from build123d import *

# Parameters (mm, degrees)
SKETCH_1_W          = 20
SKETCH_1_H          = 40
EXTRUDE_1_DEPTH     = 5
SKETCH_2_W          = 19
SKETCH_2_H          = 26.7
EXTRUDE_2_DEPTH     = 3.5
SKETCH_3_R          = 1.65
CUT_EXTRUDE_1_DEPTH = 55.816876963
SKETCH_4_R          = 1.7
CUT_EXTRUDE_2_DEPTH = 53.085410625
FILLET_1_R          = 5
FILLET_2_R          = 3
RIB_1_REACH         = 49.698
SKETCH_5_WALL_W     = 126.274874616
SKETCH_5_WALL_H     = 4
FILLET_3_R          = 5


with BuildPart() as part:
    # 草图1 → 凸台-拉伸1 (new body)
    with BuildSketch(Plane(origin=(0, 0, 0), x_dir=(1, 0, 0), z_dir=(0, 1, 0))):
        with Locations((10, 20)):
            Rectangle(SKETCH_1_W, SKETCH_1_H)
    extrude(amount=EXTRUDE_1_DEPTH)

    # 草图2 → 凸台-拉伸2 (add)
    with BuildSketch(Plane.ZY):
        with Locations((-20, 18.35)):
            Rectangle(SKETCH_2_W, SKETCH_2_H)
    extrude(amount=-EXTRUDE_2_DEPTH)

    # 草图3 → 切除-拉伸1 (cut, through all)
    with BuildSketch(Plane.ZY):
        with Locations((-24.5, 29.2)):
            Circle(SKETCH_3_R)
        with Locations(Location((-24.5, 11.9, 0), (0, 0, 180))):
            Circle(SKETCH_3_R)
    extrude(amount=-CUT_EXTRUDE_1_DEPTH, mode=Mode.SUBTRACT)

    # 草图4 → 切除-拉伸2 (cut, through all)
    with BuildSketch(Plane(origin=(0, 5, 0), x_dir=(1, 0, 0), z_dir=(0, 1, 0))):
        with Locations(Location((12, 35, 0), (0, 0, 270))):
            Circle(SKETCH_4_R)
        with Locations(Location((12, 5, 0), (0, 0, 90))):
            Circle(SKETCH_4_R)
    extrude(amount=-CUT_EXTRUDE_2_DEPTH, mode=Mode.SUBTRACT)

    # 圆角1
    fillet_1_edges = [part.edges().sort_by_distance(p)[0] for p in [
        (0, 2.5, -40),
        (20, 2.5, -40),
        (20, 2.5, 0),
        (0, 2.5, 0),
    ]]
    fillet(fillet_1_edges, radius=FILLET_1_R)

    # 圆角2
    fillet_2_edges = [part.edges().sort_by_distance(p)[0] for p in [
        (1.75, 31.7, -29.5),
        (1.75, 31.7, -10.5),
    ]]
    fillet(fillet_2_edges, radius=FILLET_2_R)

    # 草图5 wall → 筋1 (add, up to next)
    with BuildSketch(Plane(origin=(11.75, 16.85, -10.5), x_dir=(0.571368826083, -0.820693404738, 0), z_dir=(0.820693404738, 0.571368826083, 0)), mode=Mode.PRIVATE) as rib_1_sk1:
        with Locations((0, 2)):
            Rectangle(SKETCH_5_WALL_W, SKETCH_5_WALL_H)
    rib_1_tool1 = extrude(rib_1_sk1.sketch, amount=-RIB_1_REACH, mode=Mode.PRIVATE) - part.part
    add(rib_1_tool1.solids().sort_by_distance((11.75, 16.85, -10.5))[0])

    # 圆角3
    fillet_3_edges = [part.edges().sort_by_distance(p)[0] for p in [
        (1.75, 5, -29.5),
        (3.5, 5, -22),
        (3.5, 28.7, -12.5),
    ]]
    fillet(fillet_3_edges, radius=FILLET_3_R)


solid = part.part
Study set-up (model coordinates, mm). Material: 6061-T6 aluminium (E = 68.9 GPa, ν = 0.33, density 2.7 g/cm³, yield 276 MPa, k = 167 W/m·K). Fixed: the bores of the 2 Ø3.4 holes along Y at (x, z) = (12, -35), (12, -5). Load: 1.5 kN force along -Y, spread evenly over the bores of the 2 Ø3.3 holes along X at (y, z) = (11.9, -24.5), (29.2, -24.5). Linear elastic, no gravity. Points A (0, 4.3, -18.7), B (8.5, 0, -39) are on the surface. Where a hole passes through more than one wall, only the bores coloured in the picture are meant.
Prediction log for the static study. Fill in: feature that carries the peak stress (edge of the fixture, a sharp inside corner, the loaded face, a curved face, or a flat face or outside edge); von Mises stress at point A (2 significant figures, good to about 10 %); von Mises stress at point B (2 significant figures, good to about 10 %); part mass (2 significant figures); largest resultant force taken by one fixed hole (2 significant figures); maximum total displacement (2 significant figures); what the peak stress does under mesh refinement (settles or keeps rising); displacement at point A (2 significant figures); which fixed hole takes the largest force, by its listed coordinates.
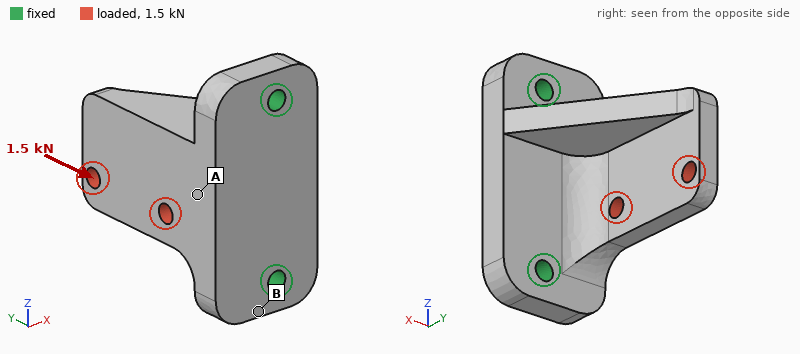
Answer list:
edge of the fixture
35 MPa
75 MPa
17 g
1.0 kN
0.12 mm
keeps rising
0.047 mm
(12, -35)
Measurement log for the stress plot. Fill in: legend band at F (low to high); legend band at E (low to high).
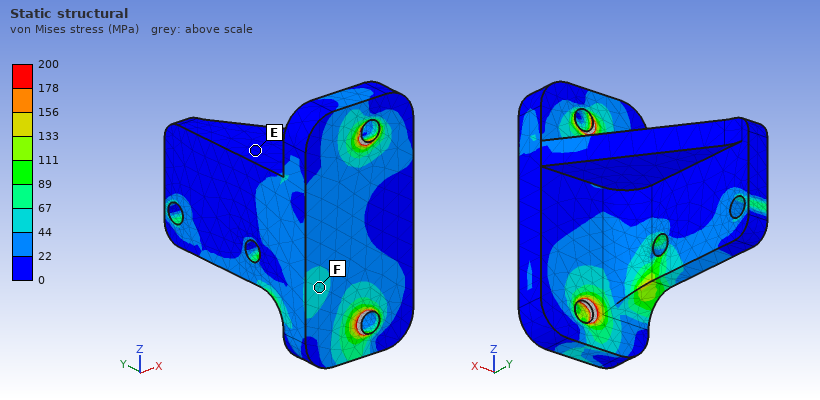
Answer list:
44 to 67 MPa
0 to 22 MPa
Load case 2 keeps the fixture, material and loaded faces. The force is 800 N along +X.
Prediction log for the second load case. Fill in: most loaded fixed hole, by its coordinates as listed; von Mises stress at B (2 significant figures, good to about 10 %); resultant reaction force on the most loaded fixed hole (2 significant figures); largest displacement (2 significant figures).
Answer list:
(12, -35)
50 MPa
520 N
0.31 mm
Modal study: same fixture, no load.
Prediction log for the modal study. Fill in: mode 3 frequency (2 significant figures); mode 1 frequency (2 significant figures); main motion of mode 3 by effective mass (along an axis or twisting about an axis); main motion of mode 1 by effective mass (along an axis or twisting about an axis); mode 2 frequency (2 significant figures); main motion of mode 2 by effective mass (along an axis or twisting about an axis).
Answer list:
13 kHz
5600 Hz
along Y
along X
10 kHz
along Z
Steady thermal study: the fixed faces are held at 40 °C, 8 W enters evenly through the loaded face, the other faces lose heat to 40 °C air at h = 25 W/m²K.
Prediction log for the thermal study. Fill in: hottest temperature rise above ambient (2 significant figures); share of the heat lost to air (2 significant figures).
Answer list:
15 K
4.6 %
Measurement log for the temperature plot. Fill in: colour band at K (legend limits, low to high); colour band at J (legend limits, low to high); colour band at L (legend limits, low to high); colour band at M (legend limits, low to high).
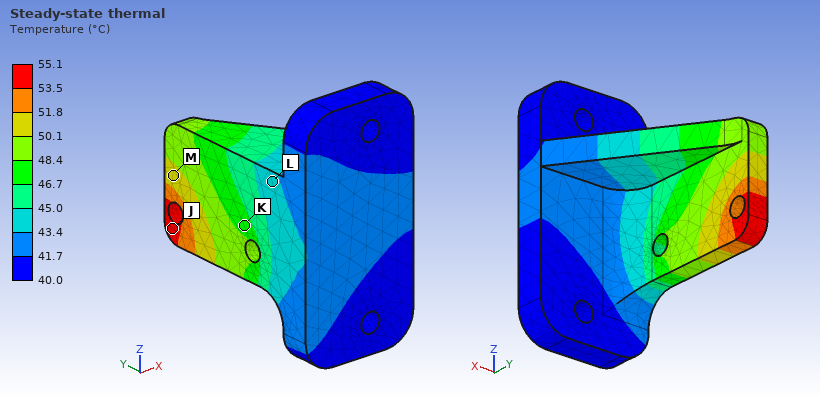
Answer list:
46.7 to 48.4 °C
53.5 to 55.1 °C
43.4 to 45.0 °C
50.1 to 51.8 °C
